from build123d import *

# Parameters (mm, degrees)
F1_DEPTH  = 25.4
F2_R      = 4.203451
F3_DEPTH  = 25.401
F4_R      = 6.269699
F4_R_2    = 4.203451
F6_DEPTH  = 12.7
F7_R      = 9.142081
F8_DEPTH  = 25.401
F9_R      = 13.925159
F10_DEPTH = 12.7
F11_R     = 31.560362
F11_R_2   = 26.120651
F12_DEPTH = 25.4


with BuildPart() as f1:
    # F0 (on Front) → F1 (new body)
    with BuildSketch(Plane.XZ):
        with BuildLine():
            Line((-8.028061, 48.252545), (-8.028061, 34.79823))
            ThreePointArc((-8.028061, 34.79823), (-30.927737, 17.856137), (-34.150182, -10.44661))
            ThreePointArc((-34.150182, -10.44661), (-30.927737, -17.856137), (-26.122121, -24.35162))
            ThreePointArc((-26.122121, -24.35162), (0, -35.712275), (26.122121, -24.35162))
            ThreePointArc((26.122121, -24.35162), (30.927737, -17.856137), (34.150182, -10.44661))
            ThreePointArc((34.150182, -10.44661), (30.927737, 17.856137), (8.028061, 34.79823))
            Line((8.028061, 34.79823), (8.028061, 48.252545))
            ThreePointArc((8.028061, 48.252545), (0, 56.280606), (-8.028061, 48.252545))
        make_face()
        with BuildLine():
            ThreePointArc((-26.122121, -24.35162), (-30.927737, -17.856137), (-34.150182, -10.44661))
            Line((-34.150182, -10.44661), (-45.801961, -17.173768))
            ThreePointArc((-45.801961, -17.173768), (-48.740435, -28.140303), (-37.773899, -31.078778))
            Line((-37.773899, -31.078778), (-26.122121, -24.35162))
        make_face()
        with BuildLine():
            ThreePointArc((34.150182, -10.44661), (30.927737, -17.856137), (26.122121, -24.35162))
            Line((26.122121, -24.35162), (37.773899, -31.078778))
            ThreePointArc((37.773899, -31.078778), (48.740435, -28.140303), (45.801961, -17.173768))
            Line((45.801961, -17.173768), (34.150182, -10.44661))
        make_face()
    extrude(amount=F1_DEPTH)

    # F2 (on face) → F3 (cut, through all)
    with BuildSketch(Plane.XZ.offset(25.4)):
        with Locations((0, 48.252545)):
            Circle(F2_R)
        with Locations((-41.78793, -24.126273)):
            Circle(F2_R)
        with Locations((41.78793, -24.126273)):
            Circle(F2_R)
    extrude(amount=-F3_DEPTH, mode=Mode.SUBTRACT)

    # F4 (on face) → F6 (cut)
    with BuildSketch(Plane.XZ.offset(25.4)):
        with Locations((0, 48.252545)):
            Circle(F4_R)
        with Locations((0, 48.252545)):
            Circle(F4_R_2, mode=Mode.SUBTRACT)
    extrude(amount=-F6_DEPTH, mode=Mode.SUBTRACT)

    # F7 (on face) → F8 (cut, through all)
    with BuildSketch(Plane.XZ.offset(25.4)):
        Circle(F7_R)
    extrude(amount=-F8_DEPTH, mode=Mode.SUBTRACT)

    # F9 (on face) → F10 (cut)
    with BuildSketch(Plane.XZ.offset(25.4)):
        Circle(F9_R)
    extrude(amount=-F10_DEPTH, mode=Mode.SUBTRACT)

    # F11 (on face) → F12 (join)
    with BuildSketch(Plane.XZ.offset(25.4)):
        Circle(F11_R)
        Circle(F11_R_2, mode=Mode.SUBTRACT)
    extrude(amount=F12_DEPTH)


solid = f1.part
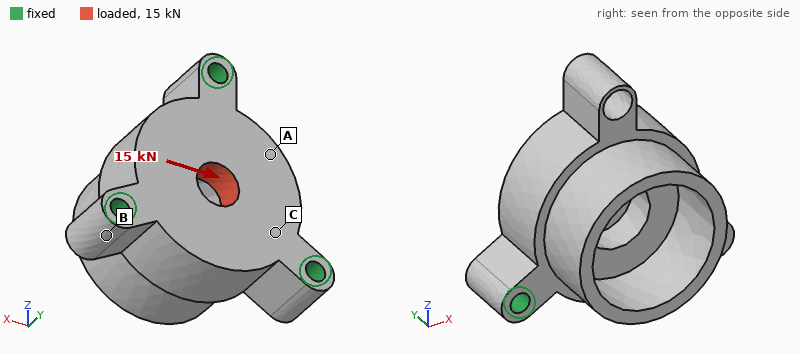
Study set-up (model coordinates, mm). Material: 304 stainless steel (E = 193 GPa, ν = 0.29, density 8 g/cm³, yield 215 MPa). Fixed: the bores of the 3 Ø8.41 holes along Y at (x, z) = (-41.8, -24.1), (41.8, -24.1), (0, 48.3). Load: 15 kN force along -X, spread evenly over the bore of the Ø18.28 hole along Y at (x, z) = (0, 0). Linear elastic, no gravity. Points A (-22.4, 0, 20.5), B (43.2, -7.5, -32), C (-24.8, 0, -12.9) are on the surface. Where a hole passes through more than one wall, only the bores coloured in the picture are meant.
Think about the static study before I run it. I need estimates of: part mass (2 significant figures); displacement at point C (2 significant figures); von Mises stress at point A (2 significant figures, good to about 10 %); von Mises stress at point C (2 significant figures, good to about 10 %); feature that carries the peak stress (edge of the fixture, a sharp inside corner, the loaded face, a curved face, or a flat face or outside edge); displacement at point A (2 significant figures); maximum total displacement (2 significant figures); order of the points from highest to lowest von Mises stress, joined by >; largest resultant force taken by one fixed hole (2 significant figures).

1.1 kg
2.4 µm
7.7 MPa
22 MPa
edge of the fixture
5.1 µm
6.3 µm
C > A > B
6.8 kN
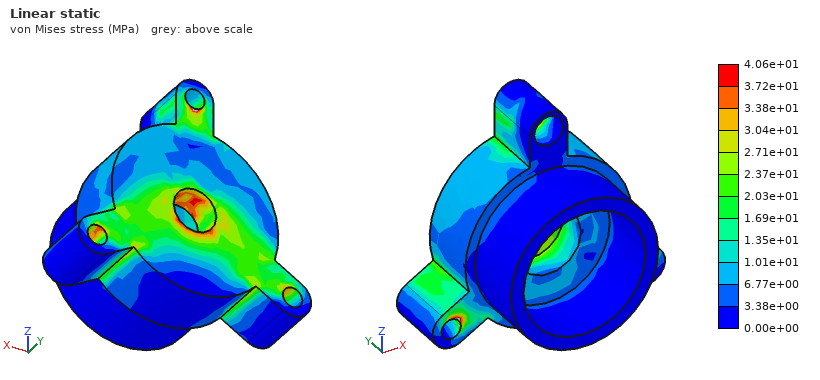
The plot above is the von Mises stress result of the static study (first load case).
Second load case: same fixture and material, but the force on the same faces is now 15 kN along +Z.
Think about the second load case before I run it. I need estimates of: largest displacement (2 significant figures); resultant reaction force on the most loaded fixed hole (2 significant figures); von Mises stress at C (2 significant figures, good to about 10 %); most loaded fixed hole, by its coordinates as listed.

7.3 µm
5.9 kN
13 MPa
(0, 48.3)
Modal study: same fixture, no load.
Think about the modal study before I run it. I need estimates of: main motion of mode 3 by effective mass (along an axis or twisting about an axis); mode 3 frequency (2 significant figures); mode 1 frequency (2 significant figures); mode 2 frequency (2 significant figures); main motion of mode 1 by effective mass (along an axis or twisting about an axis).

along Y
8500 Hz
7200 Hz
7500 Hz
along X
